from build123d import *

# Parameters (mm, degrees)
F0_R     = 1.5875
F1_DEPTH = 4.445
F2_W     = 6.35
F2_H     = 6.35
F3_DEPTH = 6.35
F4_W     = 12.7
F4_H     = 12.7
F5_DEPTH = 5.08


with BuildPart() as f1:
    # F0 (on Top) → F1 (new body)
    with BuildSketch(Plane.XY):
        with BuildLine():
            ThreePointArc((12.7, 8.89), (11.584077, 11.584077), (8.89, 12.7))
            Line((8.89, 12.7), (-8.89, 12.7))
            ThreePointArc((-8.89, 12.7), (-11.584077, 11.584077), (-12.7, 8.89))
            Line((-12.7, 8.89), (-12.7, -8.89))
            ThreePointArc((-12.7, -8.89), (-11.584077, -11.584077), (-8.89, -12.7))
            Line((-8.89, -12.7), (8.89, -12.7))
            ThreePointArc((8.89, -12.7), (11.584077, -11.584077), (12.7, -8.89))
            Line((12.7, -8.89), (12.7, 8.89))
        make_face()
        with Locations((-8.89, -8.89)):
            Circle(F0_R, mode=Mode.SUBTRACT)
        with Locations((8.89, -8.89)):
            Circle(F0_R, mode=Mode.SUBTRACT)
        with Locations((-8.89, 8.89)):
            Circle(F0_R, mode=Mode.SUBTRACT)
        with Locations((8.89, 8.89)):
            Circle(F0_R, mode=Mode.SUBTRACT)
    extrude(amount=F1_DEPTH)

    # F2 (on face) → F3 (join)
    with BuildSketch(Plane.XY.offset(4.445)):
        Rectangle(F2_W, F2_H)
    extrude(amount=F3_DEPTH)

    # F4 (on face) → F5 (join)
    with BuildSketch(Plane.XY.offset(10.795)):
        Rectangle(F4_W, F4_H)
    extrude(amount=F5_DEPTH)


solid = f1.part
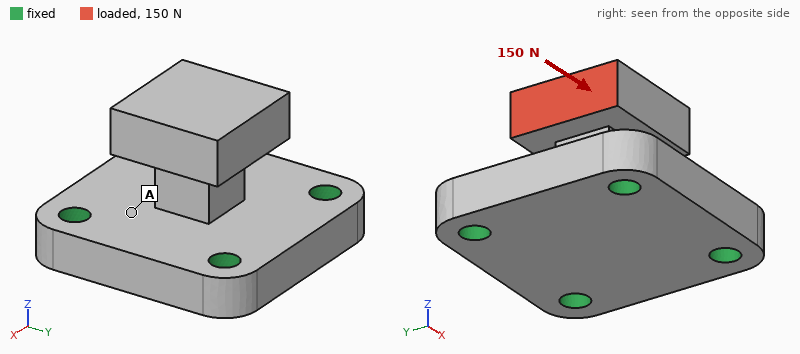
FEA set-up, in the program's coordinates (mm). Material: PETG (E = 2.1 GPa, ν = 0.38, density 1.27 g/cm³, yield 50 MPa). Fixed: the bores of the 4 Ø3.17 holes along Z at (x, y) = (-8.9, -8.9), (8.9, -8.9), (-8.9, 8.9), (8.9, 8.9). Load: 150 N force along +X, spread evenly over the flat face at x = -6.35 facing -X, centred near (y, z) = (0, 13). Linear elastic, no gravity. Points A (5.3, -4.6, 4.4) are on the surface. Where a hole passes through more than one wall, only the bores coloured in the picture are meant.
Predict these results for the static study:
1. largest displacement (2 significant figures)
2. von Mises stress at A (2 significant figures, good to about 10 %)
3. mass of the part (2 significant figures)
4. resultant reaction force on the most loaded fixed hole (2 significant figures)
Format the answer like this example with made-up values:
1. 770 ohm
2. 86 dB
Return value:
1. 0.44 mm
2. 4.6 MPa
3. 4.8 g
4. 70 N
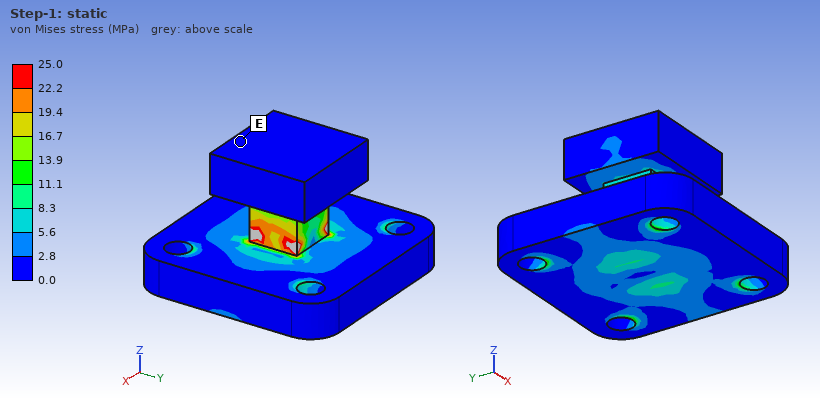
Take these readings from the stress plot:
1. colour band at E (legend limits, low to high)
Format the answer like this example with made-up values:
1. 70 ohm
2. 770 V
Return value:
1. 0.0 to 2.8 MPa
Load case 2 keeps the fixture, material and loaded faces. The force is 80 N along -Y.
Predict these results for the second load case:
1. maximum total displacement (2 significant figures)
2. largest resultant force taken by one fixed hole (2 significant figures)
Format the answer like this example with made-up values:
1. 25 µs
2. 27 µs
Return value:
1. 0.40 mm
2. 40 N
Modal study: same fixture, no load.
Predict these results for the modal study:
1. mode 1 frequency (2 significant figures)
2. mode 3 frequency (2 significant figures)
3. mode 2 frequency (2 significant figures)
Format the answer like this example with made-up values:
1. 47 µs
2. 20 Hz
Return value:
1. 3100 Hz
2. 4400 Hz
3. 3200 Hz
